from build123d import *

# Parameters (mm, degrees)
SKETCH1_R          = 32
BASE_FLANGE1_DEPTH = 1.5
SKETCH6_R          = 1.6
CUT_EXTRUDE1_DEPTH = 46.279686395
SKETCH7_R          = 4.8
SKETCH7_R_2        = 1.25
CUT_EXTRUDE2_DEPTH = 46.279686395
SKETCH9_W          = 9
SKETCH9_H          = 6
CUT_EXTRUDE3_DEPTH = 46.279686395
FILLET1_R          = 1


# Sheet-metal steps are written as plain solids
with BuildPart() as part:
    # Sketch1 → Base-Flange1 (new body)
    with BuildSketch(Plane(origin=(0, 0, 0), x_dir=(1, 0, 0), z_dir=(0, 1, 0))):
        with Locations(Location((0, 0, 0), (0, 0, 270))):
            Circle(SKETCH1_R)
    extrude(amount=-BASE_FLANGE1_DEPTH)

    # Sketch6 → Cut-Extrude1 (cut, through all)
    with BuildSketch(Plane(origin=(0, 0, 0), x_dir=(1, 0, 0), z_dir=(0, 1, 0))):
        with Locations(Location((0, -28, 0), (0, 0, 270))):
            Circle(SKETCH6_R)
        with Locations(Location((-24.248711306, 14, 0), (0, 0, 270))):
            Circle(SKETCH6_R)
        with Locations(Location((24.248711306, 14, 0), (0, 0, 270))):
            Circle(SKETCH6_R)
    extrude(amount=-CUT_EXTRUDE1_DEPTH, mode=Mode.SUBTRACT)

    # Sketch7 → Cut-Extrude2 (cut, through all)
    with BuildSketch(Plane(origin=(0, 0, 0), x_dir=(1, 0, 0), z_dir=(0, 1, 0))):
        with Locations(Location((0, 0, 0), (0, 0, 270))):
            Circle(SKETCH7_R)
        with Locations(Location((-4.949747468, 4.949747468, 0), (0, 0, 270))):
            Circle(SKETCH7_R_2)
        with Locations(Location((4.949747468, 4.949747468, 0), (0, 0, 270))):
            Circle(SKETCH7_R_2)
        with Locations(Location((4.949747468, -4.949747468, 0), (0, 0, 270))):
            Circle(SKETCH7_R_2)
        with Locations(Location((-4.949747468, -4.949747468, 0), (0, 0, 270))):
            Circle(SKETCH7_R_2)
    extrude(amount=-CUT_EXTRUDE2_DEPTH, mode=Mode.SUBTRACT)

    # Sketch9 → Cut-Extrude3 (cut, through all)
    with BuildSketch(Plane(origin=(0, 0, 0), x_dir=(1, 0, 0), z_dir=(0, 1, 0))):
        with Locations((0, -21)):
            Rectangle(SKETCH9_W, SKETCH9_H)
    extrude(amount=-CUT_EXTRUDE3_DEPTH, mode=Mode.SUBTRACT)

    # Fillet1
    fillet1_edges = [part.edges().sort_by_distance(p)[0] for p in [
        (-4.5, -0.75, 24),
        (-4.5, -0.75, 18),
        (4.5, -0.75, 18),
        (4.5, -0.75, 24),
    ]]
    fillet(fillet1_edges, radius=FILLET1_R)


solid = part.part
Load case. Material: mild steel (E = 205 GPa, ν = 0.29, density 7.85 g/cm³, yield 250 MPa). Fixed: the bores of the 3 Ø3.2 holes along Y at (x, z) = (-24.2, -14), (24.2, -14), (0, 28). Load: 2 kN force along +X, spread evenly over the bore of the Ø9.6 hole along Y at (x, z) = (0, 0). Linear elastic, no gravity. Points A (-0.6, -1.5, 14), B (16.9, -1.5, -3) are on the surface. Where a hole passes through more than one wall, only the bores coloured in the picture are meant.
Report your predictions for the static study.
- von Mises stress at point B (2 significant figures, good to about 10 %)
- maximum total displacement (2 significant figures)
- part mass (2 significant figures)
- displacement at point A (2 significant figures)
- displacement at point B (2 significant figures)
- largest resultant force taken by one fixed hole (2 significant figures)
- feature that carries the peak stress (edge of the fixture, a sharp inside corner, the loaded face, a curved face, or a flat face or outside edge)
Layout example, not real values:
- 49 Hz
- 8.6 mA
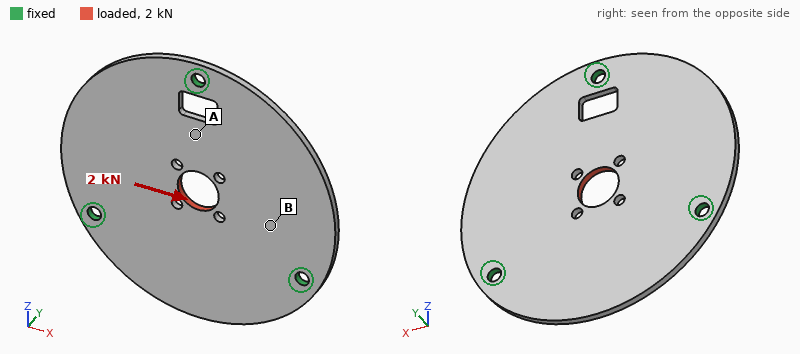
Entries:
- 29 MPa
- 6.9 µm
- 36 g
- 3.6 µm
- 3.3 µm
- 730 N
- a curved face
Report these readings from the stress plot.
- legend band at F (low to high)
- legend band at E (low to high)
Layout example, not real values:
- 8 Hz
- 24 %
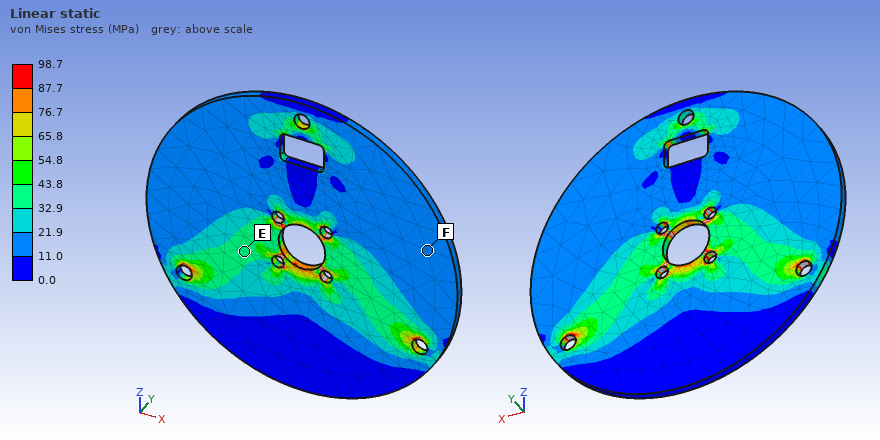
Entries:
- 11.0 to 21.9 MPa
- 32.9 to 43.8 MPa
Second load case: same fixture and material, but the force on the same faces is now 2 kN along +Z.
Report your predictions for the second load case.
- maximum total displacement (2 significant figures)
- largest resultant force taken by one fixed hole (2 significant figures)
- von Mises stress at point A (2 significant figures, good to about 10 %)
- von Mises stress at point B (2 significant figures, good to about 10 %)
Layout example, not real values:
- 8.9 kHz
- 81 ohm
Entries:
- 7.2 µm
- 790 N
- 26 MPa
- 21 MPa
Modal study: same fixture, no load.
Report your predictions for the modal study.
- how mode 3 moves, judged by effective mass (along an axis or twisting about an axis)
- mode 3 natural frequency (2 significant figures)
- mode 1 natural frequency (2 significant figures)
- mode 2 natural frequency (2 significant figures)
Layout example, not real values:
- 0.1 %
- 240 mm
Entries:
- along Y
- 2600 Hz
- 2400 Hz
- 2400 Hz
